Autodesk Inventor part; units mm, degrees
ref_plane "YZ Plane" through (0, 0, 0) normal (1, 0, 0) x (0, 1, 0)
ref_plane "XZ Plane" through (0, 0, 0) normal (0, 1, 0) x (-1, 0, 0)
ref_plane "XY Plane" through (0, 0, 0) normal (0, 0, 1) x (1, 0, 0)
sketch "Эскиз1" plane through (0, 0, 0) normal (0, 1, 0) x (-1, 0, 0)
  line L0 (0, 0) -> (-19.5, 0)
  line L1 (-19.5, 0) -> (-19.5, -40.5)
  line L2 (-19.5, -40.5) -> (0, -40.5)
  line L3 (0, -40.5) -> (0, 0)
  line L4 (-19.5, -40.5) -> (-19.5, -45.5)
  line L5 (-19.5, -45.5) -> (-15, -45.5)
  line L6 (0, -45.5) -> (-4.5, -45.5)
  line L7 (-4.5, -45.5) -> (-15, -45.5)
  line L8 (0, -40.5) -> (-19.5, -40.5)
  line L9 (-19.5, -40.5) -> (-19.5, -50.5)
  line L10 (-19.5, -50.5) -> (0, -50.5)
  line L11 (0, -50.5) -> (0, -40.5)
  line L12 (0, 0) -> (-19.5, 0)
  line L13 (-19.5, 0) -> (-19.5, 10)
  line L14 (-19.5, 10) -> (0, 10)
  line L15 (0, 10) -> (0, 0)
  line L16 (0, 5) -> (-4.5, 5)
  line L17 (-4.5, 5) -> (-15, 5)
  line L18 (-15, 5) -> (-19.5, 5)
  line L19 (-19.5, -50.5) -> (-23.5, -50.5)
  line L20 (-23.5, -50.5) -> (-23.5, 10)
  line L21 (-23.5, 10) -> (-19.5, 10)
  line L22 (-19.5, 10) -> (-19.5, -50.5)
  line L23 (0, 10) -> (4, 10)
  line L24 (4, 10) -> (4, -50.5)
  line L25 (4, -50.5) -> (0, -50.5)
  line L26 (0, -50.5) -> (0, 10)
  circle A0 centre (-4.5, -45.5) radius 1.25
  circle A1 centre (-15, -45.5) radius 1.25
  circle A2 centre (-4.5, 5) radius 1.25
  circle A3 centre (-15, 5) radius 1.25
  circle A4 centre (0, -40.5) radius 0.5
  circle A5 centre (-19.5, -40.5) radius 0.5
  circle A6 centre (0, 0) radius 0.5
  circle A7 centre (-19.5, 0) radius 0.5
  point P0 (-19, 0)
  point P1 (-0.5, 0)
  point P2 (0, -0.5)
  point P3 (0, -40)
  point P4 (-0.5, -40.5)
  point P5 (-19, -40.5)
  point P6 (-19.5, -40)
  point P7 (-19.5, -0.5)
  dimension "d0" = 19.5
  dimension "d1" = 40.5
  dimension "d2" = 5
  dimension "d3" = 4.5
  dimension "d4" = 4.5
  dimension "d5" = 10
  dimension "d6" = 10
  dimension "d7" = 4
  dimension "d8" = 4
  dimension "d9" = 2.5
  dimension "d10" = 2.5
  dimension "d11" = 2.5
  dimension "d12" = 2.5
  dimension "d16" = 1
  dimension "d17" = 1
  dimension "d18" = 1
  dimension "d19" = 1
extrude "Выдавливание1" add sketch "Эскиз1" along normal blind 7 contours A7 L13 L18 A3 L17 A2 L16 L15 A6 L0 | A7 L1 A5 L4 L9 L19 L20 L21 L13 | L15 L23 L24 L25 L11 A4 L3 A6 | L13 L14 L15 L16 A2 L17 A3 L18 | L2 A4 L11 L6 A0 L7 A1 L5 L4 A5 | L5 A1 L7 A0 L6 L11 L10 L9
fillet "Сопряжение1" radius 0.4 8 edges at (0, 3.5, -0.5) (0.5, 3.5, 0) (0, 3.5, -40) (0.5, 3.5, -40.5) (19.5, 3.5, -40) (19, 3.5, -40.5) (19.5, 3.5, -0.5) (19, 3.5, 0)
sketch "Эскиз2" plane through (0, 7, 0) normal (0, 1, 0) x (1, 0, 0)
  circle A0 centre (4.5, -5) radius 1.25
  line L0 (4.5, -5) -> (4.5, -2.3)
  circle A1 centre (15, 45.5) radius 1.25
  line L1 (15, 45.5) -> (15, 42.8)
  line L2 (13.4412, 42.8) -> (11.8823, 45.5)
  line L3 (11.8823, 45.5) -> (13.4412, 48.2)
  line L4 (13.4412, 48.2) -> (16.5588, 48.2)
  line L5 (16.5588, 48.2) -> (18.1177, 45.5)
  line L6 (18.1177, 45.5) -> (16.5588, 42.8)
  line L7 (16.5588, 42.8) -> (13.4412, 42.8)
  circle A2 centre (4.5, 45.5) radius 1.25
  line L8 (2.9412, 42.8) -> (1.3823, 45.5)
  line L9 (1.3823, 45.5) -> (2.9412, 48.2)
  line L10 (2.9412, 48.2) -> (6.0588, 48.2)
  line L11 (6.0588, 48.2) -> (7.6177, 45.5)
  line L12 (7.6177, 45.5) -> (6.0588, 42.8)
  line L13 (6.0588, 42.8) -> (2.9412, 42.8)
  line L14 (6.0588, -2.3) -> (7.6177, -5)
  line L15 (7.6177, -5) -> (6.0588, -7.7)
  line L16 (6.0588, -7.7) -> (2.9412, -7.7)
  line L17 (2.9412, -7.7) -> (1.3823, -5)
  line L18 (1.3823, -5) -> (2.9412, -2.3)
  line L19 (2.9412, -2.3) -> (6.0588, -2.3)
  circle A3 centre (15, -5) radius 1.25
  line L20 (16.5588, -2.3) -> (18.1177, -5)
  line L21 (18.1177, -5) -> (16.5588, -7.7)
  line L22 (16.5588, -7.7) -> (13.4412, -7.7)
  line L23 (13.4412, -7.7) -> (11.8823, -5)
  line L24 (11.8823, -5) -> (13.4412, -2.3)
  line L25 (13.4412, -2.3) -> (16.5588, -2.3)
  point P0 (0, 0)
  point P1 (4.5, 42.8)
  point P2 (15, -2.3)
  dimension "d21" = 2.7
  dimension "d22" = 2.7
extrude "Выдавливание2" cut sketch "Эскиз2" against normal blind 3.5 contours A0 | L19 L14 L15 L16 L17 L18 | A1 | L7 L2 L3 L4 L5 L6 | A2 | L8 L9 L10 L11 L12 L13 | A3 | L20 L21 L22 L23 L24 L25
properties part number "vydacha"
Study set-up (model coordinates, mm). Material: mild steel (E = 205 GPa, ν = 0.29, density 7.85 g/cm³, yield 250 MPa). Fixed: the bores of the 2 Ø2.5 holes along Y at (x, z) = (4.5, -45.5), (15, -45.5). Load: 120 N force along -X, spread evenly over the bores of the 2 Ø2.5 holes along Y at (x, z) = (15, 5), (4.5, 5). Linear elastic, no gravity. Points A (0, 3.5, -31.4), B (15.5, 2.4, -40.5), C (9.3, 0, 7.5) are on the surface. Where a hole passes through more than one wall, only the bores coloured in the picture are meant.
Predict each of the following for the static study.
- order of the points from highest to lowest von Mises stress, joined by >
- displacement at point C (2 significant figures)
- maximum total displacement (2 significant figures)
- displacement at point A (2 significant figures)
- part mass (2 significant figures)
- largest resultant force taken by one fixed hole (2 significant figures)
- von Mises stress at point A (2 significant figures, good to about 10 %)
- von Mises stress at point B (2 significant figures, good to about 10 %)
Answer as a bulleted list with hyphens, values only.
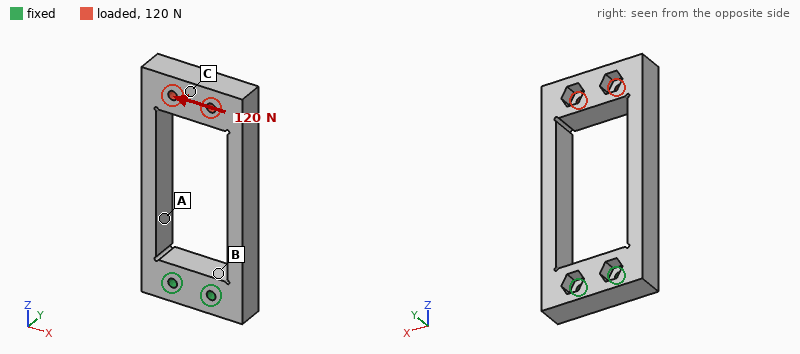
- A > B > C
- 86 µm
- 87 µm
- 16 µm
- 45 g
- 440 N
- 32 MPa
- 21 MPa
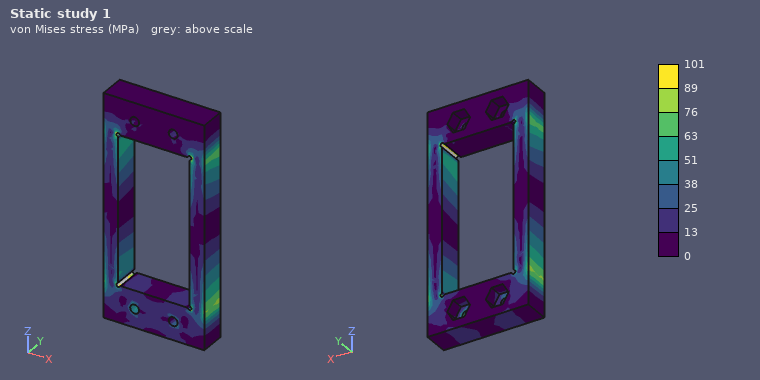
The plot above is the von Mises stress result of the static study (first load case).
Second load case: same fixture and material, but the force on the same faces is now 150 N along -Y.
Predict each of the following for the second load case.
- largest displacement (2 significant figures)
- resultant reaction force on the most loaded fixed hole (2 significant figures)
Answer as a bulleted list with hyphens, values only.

- 0.21 mm
- 99 N
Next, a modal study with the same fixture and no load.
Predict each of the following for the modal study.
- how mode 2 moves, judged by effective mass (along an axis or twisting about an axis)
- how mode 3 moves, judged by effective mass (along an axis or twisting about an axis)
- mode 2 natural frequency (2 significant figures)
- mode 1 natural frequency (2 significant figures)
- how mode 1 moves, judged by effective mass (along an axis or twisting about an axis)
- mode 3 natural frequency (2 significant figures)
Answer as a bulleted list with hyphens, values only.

- along X
- twisting about Z
- 1400 Hz
- 1100 Hz
- along Y
- 3100 Hz
